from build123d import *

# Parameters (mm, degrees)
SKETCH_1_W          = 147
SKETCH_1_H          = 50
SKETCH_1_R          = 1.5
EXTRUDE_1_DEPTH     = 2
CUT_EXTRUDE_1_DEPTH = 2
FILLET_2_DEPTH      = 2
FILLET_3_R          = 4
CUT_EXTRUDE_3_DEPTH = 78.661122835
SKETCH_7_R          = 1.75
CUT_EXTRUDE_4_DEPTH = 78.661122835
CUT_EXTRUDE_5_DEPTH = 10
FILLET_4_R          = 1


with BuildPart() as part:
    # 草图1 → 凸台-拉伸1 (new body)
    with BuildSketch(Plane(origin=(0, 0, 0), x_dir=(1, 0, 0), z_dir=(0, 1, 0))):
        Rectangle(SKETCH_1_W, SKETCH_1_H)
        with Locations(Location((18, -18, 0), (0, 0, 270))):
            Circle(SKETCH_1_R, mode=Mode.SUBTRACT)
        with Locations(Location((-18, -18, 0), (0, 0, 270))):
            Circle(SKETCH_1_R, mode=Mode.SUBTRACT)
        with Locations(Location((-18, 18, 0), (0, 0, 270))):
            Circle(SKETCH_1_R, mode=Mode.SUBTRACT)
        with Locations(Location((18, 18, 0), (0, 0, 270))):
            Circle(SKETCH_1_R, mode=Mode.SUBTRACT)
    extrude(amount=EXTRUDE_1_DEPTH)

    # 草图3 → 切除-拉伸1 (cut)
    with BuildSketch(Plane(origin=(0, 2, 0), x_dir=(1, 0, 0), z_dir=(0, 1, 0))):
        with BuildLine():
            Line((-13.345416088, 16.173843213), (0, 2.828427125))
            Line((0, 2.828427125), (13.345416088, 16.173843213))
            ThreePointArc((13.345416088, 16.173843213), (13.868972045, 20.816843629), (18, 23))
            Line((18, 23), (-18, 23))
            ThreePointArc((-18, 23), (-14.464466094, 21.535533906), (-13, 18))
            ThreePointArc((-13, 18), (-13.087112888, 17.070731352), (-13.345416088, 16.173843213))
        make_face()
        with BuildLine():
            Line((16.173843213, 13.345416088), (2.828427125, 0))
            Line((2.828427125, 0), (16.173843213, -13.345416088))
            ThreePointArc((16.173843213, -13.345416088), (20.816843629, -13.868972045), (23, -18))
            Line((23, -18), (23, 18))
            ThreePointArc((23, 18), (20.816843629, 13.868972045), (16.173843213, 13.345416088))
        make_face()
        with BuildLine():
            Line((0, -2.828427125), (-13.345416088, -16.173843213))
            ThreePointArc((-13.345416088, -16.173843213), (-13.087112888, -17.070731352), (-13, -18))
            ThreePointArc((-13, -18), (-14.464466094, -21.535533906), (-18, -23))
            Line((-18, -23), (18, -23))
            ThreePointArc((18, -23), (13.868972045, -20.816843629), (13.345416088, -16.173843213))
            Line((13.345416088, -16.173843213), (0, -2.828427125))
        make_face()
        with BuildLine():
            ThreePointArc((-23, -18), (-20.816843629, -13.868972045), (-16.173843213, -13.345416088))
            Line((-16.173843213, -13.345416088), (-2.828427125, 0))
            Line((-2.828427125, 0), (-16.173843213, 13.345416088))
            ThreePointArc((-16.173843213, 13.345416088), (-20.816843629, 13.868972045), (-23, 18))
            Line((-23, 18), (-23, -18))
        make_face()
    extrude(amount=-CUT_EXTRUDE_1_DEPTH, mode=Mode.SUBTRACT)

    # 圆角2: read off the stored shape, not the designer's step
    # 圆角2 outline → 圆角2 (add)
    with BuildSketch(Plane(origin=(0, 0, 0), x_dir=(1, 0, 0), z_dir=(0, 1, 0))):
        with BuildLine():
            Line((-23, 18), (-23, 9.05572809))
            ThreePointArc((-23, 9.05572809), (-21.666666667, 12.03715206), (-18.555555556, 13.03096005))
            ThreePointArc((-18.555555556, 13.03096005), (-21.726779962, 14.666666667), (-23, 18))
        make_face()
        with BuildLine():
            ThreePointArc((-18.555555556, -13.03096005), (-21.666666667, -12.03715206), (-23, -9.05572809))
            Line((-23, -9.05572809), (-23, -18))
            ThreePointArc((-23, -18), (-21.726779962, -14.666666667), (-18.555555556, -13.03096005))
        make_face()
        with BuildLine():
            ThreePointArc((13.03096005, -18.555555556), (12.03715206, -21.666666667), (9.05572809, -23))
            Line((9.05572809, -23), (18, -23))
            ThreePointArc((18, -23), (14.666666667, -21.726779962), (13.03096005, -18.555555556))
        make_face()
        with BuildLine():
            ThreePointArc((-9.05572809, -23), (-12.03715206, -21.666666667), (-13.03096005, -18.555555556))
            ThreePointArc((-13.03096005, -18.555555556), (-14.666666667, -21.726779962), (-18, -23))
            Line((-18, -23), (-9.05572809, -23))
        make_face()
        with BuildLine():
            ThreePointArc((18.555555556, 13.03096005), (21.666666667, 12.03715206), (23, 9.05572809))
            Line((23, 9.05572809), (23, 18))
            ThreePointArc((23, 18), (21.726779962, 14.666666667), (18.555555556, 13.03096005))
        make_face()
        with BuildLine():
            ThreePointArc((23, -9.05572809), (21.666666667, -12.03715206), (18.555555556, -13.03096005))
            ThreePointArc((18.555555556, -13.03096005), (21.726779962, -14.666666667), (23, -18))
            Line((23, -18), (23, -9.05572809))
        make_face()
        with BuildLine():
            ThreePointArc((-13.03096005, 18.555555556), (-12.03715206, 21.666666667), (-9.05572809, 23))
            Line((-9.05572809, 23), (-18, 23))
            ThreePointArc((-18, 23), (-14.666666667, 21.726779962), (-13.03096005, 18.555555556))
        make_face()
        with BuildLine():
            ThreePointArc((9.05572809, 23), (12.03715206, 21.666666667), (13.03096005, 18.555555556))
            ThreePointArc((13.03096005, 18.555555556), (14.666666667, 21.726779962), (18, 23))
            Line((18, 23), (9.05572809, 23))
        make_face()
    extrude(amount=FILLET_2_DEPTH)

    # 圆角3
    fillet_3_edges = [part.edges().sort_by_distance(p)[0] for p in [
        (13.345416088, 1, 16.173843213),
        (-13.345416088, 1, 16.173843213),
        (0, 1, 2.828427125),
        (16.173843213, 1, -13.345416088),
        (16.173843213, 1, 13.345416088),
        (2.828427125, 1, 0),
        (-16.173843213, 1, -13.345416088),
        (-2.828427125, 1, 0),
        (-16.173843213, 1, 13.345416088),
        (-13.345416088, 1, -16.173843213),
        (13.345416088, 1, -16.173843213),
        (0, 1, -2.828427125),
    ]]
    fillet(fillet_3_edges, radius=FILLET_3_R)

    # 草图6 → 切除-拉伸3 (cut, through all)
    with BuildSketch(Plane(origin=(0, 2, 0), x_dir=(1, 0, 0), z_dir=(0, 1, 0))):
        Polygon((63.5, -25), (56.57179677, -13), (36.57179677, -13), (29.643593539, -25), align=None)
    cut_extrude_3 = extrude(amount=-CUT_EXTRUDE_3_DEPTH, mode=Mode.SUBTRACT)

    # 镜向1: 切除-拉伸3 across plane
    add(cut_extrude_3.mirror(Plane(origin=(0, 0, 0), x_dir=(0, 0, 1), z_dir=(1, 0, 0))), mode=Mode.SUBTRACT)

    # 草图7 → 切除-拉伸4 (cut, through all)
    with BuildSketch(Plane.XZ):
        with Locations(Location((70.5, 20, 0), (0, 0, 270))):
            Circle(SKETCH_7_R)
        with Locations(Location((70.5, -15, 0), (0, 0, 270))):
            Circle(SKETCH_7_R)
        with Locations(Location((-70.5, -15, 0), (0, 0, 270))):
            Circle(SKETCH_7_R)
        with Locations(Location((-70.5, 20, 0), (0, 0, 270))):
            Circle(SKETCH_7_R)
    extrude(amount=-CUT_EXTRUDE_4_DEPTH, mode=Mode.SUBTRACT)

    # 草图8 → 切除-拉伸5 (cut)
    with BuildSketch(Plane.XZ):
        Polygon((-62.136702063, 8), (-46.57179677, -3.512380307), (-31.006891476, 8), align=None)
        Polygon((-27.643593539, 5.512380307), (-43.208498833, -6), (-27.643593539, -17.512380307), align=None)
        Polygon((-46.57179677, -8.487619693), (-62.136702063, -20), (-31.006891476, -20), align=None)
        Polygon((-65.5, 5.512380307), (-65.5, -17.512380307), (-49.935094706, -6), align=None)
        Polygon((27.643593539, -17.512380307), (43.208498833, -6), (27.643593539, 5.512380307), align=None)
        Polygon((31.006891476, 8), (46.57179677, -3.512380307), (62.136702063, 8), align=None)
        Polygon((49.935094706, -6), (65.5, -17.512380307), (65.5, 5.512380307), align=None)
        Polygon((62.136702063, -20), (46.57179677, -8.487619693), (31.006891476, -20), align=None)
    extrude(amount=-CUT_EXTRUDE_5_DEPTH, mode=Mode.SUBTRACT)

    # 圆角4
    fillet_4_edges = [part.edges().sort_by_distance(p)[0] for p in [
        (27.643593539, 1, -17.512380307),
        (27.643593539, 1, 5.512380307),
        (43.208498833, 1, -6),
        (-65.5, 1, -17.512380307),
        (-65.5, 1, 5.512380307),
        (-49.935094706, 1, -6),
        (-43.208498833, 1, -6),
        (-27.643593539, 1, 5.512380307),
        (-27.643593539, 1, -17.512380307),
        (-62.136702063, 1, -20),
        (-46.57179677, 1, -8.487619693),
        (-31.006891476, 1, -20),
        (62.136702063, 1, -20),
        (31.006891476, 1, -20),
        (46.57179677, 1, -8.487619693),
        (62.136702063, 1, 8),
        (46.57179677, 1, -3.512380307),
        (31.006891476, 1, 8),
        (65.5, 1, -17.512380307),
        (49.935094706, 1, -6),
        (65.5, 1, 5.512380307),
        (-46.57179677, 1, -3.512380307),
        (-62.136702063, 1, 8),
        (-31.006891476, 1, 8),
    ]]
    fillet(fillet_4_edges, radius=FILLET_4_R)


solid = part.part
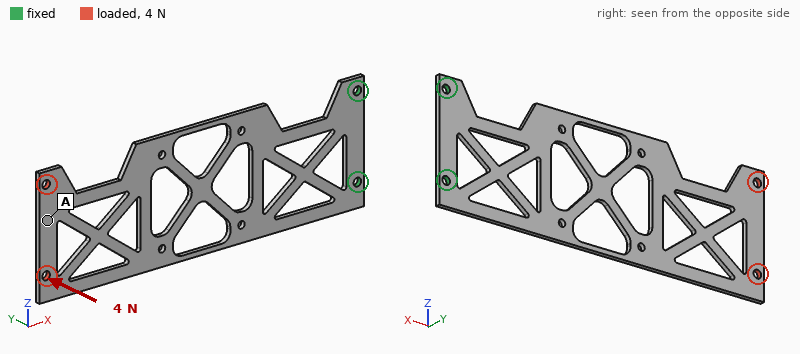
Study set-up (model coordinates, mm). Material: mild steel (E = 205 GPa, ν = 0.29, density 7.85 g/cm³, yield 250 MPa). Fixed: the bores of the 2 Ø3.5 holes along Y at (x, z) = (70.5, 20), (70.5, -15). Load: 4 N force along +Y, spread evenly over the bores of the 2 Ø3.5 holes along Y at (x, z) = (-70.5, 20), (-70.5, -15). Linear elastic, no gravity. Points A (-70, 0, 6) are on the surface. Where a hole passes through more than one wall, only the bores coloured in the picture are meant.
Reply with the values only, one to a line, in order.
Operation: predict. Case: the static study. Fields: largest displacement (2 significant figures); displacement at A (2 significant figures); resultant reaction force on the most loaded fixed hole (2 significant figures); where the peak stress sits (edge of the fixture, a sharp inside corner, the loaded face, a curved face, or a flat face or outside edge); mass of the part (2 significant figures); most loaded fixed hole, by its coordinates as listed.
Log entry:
1.7 mm
1.6 mm
2.6 N
a curved face
60 g
(70.5, 20)
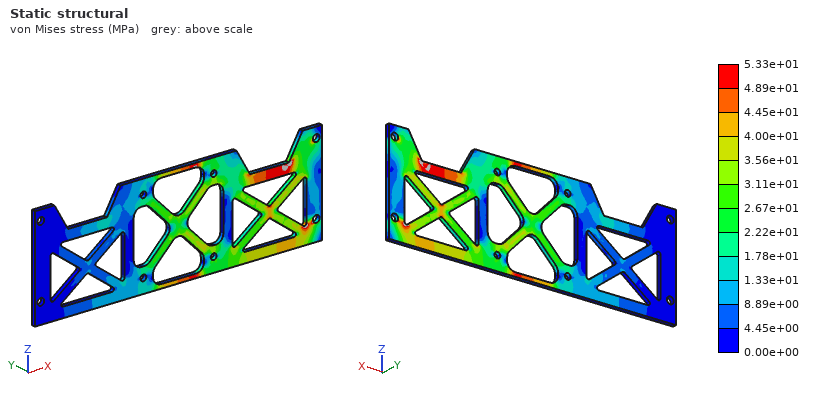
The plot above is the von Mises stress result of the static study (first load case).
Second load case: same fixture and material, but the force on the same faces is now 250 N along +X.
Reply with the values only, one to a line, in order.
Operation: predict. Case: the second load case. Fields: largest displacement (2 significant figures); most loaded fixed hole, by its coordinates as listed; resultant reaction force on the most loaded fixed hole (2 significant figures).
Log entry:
47 µm
(70.5, 20)
150 N
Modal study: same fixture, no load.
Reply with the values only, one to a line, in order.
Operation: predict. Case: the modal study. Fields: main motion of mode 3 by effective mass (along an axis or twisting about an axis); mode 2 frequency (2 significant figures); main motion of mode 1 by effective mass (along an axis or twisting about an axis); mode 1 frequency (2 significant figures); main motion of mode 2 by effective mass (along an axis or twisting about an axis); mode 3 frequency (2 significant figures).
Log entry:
along Y
350 Hz
along Y
62 Hz
twisting about X
390 Hz
